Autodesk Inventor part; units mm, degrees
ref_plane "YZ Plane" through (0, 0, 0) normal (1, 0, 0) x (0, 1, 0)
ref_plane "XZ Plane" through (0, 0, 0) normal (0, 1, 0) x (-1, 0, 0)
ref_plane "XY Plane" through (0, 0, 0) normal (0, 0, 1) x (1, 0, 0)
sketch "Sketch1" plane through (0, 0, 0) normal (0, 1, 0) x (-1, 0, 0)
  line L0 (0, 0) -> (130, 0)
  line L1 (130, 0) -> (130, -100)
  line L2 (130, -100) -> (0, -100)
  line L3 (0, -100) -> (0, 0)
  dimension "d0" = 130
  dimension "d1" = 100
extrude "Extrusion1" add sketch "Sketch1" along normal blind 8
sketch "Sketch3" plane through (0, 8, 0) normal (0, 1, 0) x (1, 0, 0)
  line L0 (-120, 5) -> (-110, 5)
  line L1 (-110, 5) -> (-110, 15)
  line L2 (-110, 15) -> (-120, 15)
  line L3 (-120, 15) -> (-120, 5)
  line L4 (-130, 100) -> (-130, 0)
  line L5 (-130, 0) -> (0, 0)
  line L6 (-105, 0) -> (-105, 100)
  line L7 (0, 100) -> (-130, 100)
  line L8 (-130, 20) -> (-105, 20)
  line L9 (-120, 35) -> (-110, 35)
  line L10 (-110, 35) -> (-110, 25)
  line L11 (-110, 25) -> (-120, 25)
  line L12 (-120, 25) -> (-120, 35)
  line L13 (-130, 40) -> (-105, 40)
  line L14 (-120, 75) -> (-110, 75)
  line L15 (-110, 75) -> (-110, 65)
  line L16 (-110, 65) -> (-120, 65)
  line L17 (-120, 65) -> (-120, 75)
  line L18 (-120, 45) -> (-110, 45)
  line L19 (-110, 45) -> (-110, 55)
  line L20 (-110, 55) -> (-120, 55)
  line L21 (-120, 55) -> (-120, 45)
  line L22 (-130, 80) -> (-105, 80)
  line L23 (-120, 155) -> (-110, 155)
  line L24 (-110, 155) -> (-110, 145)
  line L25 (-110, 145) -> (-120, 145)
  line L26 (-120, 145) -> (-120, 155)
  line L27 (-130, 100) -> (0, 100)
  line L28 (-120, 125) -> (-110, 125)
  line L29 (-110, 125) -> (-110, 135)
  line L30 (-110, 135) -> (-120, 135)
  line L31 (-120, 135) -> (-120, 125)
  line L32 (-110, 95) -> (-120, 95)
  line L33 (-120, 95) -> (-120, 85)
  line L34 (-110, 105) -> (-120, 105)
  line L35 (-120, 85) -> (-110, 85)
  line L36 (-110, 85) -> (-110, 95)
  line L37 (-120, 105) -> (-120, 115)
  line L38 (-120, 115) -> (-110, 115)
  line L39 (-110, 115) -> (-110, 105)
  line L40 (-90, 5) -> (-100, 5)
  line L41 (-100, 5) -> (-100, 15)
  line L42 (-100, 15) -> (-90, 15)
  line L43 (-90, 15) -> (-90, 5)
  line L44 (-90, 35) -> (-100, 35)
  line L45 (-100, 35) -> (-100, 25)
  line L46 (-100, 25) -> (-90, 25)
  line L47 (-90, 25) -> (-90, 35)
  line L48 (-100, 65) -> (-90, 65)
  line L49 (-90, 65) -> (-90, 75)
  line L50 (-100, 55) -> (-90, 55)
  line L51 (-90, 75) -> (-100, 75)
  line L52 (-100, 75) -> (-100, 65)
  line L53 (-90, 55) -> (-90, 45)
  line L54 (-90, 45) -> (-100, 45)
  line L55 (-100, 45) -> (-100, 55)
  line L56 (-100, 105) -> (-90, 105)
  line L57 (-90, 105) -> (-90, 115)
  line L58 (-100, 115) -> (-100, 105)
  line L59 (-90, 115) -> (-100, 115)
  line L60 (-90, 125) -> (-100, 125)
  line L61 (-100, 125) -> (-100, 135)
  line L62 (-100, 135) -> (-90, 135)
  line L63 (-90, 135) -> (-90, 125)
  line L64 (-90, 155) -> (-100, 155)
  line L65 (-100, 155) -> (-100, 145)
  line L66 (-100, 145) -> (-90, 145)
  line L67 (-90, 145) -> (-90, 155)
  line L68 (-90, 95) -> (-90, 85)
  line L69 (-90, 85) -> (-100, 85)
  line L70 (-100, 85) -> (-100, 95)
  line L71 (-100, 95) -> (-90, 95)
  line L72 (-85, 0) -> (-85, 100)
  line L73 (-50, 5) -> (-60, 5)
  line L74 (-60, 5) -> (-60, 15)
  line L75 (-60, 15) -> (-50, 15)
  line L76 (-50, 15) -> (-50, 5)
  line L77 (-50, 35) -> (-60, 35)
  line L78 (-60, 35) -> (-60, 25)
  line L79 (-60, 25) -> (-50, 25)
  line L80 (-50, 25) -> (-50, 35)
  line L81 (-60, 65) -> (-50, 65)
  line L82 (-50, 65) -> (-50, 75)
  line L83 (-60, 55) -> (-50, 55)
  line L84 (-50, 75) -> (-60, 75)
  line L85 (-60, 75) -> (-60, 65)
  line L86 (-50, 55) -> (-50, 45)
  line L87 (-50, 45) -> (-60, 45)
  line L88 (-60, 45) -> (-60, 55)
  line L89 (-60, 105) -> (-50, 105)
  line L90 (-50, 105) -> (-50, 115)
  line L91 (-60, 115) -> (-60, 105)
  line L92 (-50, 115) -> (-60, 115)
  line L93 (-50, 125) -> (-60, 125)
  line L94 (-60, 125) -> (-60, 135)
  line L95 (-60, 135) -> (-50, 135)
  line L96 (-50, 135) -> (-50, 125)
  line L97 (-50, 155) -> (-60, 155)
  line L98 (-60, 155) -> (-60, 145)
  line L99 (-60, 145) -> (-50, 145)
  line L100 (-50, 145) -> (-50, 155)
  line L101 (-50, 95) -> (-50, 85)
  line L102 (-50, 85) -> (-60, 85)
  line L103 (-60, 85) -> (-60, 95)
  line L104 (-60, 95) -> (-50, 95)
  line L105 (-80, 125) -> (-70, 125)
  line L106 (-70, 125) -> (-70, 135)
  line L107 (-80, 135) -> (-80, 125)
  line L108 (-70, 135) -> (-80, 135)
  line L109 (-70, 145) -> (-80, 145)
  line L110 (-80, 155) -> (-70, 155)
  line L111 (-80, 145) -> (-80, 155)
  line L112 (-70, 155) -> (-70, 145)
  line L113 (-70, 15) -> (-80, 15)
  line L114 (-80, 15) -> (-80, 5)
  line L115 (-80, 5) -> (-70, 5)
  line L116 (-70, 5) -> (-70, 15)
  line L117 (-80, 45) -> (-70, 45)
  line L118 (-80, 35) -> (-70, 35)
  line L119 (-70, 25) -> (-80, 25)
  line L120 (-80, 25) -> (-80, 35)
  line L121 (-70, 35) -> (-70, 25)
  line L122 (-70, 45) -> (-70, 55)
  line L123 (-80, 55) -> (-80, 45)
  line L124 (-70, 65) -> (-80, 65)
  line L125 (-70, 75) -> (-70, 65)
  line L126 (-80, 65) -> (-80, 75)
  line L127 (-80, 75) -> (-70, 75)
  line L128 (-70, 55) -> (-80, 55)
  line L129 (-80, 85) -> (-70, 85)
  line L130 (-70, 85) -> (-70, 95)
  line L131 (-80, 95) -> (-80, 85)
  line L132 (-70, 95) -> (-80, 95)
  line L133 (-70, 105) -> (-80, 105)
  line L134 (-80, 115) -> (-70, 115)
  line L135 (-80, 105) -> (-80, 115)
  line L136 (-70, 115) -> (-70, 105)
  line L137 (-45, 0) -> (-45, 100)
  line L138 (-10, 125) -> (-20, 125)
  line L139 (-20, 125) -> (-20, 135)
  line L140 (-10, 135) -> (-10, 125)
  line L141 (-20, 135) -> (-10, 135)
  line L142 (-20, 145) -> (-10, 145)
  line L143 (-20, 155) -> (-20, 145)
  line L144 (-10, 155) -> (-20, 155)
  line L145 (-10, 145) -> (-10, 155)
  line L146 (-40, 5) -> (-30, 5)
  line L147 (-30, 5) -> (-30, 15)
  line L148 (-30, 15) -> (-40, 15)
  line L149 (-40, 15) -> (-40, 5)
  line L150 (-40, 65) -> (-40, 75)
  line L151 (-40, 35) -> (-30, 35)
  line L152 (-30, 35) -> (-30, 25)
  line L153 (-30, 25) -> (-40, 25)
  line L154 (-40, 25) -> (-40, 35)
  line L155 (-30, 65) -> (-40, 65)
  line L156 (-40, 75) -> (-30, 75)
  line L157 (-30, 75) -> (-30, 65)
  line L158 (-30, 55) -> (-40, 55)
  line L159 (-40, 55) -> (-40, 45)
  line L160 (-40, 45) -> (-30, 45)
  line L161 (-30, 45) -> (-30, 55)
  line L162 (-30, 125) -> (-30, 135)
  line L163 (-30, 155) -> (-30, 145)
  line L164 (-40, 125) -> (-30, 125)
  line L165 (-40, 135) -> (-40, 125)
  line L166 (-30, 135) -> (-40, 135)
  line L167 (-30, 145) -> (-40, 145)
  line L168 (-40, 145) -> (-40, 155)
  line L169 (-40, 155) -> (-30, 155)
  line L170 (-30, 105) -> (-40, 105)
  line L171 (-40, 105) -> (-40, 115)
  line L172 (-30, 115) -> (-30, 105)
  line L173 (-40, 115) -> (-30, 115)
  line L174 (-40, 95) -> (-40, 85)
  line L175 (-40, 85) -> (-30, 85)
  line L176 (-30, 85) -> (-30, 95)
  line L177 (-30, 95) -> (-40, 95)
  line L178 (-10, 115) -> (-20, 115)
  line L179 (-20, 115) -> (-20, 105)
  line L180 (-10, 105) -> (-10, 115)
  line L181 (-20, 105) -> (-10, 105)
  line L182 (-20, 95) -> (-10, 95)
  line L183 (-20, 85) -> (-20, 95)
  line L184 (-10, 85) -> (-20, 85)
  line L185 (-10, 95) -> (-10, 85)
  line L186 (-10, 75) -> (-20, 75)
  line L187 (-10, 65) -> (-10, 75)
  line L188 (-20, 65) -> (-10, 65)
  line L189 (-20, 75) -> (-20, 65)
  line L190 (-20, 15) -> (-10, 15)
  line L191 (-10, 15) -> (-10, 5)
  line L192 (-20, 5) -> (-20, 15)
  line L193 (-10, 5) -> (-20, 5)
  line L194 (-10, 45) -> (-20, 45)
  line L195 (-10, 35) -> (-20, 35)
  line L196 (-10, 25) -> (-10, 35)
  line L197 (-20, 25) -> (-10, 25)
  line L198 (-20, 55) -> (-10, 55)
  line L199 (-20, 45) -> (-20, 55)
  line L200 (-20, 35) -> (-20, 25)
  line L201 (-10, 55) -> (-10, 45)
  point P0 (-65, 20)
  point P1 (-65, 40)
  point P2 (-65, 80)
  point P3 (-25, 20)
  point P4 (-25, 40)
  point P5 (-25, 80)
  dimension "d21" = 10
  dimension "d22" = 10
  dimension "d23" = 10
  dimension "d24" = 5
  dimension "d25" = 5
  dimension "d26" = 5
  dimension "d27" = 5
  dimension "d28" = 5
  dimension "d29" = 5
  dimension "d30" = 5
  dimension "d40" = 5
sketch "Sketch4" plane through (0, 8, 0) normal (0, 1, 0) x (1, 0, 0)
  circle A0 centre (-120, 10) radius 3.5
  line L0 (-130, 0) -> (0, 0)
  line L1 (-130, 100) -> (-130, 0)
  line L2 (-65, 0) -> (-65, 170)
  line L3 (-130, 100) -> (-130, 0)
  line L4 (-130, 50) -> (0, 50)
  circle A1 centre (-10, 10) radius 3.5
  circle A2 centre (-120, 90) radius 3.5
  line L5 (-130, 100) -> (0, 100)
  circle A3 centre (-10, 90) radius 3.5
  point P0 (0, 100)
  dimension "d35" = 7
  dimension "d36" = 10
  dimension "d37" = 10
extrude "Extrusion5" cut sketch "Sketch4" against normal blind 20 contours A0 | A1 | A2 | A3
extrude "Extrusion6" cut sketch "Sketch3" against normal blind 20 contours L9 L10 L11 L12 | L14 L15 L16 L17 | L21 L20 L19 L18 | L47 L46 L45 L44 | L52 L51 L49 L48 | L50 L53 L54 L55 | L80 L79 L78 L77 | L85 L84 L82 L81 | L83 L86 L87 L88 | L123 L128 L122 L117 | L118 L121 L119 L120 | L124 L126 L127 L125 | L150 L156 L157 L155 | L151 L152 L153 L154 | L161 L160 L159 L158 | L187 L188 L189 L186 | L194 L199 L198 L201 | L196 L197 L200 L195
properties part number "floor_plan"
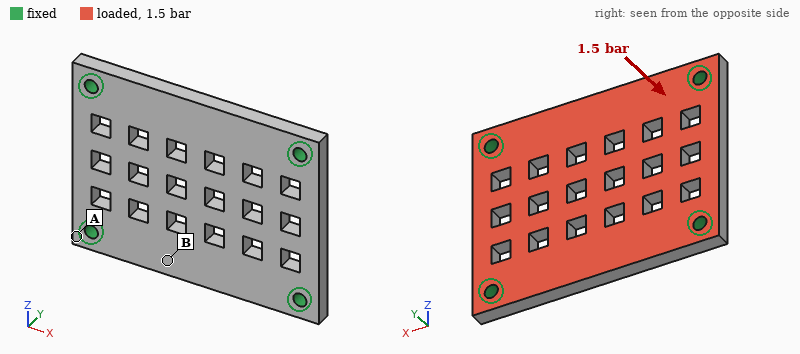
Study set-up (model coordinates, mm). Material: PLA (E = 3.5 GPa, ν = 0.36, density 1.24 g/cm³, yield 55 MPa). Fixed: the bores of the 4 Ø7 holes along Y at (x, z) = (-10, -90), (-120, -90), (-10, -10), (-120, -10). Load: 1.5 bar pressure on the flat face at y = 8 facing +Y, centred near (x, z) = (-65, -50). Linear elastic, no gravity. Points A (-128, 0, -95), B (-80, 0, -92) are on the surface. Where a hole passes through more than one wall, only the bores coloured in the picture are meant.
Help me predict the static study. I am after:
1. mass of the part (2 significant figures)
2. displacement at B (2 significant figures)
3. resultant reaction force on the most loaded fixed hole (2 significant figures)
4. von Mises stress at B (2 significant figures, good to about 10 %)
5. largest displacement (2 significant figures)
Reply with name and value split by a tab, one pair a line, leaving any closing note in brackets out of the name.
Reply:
mass of the part	110 g
displacement at B	0.43 mm
resultant reaction force on the most loaded fixed hole	410 N
von Mises stress at B	6.9 MPa
largest displacement	0.68 mm
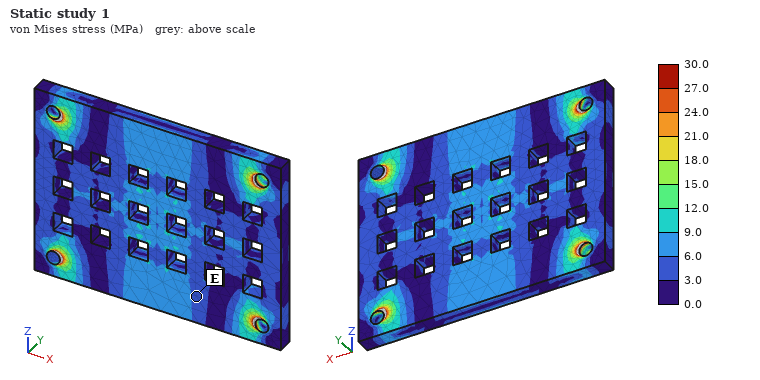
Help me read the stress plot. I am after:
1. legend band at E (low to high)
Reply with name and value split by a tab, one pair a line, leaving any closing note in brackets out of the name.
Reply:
legend band at E	3.0 to 6.0 MPa
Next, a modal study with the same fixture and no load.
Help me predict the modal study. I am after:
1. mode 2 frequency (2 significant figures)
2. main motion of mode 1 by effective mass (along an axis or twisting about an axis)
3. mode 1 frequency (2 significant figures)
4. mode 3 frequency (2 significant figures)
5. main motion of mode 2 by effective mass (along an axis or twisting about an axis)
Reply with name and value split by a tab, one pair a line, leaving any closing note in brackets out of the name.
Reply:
mode 2 frequency	1300 Hz
main motion of mode 1 by effective mass	along Y
mode 1 frequency	910 Hz
mode 3 frequency	1800 Hz
main motion of mode 2 by effective mass	twisting about X
